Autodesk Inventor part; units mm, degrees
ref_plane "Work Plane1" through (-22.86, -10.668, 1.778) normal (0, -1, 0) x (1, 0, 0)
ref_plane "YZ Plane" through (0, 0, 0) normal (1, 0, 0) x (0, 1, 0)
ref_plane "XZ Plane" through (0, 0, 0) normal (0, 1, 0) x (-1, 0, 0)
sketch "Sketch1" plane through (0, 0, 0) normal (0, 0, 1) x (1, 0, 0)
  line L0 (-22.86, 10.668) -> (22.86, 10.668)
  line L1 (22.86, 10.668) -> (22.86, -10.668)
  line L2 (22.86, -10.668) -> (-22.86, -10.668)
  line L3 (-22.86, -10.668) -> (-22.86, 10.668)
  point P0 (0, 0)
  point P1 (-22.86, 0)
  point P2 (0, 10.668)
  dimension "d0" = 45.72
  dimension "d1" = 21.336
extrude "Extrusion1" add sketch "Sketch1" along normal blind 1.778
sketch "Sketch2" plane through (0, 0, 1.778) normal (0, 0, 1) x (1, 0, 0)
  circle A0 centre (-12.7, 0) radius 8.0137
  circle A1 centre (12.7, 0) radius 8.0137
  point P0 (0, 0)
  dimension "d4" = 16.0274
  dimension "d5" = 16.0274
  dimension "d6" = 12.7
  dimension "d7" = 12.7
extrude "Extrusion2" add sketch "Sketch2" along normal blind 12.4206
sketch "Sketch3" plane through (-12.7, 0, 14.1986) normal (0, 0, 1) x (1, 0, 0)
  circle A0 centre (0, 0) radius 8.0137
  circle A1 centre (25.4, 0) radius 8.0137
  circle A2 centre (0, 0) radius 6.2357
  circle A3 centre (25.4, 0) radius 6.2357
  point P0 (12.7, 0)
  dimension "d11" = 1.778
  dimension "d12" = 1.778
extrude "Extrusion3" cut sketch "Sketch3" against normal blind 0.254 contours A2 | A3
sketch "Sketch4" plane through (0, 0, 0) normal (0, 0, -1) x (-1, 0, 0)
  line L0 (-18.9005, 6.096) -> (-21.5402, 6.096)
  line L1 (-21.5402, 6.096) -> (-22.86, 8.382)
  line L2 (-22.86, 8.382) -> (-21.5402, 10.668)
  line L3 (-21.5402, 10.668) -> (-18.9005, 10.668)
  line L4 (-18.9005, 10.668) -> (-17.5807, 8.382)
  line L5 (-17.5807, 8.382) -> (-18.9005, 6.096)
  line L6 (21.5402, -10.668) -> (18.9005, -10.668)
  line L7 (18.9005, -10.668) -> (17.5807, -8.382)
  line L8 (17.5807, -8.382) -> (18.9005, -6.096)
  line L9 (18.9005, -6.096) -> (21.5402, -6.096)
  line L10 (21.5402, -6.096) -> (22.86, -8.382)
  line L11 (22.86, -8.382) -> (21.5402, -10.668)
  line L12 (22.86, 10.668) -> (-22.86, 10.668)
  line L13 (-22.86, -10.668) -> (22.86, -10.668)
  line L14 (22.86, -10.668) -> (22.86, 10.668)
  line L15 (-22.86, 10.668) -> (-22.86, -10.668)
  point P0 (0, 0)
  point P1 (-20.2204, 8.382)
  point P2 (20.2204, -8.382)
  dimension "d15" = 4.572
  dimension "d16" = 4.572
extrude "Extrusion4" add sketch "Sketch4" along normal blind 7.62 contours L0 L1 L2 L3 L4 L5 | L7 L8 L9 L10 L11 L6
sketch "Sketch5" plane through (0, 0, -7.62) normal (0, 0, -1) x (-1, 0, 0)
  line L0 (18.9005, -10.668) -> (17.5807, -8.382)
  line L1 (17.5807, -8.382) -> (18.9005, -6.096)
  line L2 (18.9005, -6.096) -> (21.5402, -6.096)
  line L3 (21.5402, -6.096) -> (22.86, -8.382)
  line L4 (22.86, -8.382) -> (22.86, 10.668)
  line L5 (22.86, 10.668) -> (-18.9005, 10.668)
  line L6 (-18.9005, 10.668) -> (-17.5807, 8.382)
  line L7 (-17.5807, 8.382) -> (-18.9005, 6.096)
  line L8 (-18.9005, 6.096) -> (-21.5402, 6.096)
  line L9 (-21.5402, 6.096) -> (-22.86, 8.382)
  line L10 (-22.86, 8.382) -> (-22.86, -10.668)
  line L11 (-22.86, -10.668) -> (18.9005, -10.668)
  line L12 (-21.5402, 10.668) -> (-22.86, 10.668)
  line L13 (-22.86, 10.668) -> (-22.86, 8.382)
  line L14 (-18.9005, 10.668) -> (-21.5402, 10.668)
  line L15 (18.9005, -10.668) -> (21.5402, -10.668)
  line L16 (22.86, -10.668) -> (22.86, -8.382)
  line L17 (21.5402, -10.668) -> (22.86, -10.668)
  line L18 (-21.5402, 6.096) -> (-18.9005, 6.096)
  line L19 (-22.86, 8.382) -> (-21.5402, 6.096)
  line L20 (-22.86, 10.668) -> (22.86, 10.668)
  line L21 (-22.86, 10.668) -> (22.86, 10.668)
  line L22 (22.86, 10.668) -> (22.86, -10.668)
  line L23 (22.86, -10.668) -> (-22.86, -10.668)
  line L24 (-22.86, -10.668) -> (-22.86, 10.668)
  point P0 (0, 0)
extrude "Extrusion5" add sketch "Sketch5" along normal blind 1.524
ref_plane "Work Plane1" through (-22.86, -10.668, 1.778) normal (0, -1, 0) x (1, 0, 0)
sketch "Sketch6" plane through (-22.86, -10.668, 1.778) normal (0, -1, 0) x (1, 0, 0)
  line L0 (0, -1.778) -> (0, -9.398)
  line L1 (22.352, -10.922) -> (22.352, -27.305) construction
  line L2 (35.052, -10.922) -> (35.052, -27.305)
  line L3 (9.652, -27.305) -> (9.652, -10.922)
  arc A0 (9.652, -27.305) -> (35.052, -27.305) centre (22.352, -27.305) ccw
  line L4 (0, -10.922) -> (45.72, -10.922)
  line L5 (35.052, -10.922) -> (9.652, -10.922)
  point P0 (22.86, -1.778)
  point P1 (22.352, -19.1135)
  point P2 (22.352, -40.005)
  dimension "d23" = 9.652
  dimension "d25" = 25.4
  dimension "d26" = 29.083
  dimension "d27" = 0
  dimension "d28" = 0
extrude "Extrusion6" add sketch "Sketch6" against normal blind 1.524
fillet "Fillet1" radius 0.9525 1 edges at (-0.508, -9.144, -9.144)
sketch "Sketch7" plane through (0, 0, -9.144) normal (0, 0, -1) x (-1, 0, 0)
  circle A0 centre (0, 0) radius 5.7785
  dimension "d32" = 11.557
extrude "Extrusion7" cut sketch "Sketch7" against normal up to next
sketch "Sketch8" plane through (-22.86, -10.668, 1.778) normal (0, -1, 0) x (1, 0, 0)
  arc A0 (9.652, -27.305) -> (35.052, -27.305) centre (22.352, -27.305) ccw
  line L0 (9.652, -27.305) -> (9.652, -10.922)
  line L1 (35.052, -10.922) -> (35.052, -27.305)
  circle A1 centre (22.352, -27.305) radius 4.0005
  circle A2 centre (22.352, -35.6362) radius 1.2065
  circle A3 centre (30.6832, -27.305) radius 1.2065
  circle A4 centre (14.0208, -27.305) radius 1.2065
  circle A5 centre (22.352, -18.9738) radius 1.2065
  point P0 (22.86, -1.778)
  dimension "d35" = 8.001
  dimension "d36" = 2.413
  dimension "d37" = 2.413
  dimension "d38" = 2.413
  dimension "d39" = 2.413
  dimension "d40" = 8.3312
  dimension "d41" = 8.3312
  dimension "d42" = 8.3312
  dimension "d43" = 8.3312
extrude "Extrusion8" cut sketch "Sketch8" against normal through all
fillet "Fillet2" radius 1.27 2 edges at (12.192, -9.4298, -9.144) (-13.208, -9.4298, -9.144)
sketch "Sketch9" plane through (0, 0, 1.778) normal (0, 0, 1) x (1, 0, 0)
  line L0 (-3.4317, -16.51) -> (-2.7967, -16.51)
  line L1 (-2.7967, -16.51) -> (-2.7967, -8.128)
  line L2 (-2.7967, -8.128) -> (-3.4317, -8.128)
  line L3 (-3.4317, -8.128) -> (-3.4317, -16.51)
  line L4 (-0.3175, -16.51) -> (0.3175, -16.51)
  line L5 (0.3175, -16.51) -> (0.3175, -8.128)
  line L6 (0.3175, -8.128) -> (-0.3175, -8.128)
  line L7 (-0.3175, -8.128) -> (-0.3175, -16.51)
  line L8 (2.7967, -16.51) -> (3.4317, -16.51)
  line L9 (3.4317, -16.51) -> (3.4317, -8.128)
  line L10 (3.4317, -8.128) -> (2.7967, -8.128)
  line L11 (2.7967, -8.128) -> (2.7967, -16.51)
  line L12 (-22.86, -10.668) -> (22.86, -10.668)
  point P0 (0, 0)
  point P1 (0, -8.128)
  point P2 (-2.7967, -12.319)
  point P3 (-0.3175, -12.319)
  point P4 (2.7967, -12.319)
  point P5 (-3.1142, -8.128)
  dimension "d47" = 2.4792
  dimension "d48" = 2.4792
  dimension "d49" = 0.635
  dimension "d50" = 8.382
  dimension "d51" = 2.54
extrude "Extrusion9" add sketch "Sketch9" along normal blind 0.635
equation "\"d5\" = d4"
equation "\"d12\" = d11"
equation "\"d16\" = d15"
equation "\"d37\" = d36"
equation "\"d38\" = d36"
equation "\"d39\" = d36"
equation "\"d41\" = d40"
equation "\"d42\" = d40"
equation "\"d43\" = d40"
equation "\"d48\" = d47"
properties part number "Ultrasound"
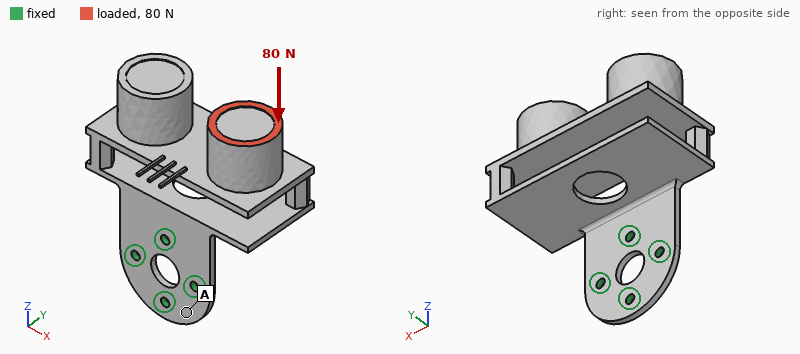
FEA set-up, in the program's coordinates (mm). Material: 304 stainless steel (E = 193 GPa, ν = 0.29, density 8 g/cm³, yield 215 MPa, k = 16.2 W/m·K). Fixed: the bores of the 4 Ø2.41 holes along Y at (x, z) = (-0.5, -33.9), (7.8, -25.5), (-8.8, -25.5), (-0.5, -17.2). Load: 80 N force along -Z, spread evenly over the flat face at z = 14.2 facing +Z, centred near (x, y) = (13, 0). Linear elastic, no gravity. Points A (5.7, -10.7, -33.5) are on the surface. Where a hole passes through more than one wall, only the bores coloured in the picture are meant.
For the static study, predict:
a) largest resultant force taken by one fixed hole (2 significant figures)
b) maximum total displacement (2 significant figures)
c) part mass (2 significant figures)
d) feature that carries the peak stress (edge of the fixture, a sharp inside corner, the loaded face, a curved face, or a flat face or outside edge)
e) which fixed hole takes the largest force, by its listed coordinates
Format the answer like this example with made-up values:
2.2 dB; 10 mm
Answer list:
81 N; 0.23 mm; 74 g; a curved face; (7.8, -25.5)
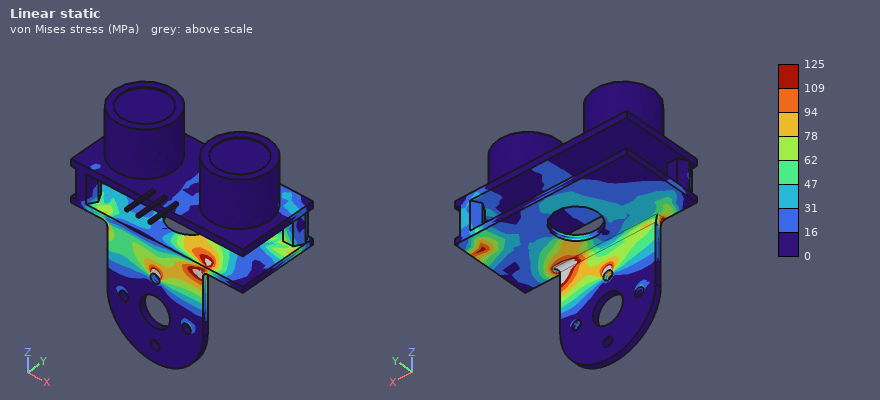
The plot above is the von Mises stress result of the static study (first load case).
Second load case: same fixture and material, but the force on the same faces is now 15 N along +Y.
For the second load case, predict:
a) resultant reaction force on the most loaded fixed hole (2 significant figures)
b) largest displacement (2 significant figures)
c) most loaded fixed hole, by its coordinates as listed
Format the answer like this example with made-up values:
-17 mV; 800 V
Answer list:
45 N; 0.15 mm; (-0.5, -17.2)
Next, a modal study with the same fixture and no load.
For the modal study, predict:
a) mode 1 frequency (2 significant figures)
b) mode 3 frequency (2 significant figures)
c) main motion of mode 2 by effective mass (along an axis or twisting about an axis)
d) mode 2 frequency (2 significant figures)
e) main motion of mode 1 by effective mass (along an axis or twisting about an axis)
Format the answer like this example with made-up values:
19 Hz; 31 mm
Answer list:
300 Hz; 680 Hz; along X; 630 Hz; along Y
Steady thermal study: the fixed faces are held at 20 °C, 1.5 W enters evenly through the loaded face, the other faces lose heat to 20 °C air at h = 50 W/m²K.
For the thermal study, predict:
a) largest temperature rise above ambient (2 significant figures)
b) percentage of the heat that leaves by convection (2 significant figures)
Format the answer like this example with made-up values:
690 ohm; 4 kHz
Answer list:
18 K; 98 %
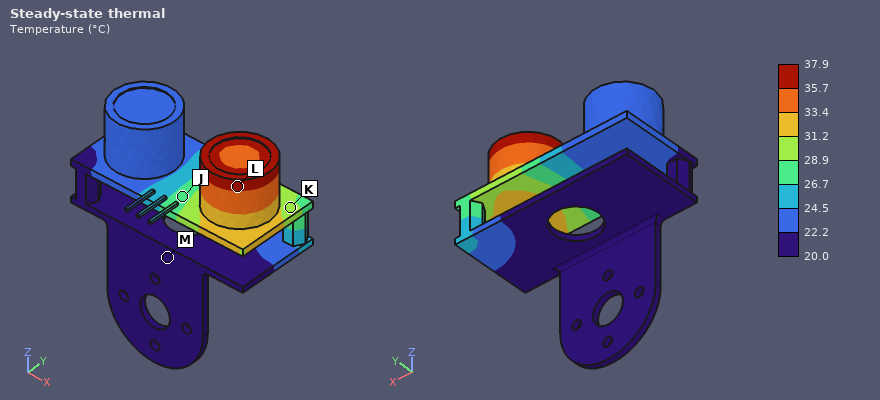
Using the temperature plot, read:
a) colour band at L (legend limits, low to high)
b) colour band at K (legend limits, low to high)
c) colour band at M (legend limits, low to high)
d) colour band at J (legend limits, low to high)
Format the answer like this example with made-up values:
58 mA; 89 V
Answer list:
35.7 to 37.9 °C; 28.9 to 31.2 °C; 20.0 to 22.2 °C; 26.7 to 28.9 °C
